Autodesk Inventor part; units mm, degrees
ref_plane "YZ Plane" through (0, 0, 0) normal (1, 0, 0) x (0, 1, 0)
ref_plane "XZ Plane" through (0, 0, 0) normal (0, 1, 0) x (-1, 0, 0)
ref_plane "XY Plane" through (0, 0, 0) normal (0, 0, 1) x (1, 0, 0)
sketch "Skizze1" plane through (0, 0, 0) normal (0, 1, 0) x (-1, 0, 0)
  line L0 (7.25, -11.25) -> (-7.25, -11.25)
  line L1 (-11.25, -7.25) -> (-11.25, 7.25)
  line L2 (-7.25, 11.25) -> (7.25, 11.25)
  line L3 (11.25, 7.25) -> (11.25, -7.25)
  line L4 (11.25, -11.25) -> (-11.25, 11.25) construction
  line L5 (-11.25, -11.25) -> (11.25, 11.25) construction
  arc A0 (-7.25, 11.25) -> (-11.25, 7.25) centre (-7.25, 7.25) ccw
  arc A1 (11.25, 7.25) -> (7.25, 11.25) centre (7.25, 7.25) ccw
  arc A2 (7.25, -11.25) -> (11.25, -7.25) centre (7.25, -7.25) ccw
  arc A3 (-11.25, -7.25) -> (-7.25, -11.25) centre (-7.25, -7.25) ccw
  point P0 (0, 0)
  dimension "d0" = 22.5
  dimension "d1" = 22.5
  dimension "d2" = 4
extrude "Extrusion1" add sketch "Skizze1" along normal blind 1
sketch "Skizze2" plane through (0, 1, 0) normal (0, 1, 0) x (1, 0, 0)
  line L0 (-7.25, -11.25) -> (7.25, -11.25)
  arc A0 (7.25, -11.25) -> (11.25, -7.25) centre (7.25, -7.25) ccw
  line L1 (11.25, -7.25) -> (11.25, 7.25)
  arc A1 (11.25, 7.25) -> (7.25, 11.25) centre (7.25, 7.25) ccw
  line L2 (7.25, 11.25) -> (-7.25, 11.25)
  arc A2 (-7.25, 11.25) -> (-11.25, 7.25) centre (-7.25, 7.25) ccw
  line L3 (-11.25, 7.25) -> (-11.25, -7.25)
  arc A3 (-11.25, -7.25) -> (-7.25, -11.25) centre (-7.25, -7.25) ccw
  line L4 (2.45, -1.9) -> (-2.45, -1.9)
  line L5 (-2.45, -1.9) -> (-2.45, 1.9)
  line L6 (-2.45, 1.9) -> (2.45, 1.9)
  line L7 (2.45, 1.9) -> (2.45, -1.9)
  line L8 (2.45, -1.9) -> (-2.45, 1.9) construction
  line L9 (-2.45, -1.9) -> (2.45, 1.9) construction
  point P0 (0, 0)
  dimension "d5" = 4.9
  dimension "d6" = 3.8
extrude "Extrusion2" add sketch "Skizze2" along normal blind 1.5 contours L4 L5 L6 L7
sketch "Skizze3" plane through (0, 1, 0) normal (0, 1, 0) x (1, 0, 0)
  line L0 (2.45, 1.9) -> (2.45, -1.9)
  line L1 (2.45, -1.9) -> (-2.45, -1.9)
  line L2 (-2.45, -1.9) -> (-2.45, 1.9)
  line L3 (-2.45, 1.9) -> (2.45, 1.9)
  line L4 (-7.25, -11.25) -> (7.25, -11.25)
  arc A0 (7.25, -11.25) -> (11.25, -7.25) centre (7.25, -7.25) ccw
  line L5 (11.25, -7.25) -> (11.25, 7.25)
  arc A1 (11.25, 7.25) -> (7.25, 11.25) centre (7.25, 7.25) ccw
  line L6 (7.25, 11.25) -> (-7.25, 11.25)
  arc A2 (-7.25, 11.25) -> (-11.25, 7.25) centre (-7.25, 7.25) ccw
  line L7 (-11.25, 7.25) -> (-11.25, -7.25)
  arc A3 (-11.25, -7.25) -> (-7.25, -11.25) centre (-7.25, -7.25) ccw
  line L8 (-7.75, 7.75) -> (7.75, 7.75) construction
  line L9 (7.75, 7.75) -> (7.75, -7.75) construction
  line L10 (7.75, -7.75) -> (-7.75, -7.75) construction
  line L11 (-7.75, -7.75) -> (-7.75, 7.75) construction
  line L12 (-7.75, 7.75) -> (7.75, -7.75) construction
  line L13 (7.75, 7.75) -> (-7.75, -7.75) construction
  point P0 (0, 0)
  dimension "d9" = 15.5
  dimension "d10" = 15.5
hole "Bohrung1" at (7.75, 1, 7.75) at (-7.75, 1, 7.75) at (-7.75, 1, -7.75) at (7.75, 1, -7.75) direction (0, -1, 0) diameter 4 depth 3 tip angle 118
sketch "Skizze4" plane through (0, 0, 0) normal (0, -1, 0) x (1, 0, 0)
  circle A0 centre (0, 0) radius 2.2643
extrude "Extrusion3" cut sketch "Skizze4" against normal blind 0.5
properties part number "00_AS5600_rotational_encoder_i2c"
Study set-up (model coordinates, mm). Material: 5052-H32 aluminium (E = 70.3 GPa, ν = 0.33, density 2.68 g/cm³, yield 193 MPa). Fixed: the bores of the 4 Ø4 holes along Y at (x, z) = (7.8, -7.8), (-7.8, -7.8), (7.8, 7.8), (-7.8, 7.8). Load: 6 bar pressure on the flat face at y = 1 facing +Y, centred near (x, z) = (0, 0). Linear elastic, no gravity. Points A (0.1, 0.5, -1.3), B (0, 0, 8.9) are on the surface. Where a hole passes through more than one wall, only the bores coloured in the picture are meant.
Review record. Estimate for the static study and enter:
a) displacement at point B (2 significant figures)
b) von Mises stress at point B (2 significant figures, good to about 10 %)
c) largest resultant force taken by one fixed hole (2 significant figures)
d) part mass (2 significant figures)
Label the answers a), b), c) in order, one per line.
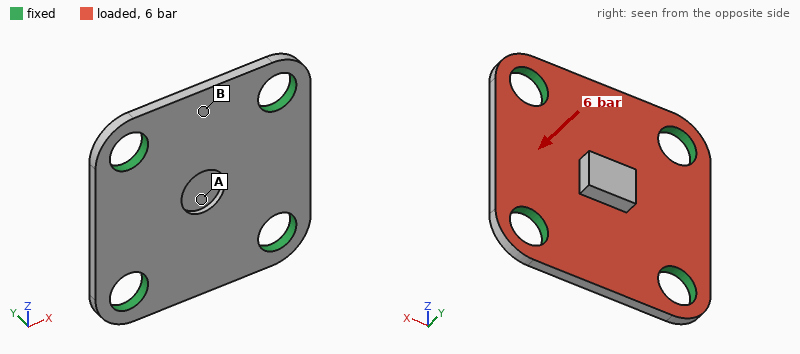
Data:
a) 6.6 µm
b) 23 MPa
c) 64 N
d) 1.2 g
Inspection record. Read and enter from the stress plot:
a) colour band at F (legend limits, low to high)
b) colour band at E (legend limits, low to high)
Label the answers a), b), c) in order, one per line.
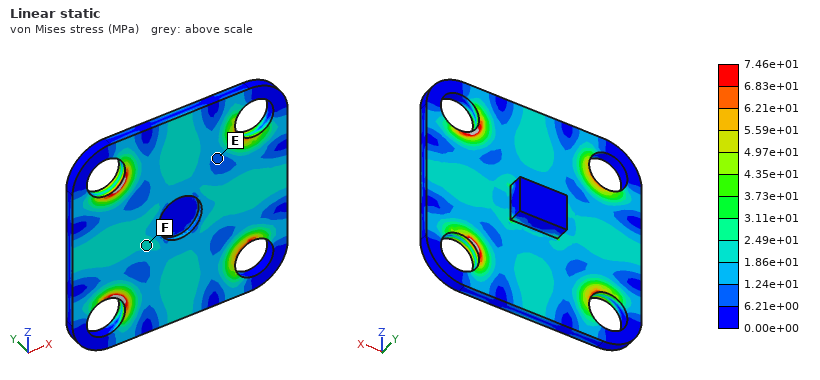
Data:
a) 1.86e+01 to 2.49e+01 MPa
b) 6.21e+00 to 1.24e+01 MPa
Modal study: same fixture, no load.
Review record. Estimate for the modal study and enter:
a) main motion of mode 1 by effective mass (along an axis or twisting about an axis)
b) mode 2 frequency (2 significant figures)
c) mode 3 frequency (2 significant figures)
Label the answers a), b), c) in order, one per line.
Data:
a) along Y
b) 34 kHz
c) 34 kHz
